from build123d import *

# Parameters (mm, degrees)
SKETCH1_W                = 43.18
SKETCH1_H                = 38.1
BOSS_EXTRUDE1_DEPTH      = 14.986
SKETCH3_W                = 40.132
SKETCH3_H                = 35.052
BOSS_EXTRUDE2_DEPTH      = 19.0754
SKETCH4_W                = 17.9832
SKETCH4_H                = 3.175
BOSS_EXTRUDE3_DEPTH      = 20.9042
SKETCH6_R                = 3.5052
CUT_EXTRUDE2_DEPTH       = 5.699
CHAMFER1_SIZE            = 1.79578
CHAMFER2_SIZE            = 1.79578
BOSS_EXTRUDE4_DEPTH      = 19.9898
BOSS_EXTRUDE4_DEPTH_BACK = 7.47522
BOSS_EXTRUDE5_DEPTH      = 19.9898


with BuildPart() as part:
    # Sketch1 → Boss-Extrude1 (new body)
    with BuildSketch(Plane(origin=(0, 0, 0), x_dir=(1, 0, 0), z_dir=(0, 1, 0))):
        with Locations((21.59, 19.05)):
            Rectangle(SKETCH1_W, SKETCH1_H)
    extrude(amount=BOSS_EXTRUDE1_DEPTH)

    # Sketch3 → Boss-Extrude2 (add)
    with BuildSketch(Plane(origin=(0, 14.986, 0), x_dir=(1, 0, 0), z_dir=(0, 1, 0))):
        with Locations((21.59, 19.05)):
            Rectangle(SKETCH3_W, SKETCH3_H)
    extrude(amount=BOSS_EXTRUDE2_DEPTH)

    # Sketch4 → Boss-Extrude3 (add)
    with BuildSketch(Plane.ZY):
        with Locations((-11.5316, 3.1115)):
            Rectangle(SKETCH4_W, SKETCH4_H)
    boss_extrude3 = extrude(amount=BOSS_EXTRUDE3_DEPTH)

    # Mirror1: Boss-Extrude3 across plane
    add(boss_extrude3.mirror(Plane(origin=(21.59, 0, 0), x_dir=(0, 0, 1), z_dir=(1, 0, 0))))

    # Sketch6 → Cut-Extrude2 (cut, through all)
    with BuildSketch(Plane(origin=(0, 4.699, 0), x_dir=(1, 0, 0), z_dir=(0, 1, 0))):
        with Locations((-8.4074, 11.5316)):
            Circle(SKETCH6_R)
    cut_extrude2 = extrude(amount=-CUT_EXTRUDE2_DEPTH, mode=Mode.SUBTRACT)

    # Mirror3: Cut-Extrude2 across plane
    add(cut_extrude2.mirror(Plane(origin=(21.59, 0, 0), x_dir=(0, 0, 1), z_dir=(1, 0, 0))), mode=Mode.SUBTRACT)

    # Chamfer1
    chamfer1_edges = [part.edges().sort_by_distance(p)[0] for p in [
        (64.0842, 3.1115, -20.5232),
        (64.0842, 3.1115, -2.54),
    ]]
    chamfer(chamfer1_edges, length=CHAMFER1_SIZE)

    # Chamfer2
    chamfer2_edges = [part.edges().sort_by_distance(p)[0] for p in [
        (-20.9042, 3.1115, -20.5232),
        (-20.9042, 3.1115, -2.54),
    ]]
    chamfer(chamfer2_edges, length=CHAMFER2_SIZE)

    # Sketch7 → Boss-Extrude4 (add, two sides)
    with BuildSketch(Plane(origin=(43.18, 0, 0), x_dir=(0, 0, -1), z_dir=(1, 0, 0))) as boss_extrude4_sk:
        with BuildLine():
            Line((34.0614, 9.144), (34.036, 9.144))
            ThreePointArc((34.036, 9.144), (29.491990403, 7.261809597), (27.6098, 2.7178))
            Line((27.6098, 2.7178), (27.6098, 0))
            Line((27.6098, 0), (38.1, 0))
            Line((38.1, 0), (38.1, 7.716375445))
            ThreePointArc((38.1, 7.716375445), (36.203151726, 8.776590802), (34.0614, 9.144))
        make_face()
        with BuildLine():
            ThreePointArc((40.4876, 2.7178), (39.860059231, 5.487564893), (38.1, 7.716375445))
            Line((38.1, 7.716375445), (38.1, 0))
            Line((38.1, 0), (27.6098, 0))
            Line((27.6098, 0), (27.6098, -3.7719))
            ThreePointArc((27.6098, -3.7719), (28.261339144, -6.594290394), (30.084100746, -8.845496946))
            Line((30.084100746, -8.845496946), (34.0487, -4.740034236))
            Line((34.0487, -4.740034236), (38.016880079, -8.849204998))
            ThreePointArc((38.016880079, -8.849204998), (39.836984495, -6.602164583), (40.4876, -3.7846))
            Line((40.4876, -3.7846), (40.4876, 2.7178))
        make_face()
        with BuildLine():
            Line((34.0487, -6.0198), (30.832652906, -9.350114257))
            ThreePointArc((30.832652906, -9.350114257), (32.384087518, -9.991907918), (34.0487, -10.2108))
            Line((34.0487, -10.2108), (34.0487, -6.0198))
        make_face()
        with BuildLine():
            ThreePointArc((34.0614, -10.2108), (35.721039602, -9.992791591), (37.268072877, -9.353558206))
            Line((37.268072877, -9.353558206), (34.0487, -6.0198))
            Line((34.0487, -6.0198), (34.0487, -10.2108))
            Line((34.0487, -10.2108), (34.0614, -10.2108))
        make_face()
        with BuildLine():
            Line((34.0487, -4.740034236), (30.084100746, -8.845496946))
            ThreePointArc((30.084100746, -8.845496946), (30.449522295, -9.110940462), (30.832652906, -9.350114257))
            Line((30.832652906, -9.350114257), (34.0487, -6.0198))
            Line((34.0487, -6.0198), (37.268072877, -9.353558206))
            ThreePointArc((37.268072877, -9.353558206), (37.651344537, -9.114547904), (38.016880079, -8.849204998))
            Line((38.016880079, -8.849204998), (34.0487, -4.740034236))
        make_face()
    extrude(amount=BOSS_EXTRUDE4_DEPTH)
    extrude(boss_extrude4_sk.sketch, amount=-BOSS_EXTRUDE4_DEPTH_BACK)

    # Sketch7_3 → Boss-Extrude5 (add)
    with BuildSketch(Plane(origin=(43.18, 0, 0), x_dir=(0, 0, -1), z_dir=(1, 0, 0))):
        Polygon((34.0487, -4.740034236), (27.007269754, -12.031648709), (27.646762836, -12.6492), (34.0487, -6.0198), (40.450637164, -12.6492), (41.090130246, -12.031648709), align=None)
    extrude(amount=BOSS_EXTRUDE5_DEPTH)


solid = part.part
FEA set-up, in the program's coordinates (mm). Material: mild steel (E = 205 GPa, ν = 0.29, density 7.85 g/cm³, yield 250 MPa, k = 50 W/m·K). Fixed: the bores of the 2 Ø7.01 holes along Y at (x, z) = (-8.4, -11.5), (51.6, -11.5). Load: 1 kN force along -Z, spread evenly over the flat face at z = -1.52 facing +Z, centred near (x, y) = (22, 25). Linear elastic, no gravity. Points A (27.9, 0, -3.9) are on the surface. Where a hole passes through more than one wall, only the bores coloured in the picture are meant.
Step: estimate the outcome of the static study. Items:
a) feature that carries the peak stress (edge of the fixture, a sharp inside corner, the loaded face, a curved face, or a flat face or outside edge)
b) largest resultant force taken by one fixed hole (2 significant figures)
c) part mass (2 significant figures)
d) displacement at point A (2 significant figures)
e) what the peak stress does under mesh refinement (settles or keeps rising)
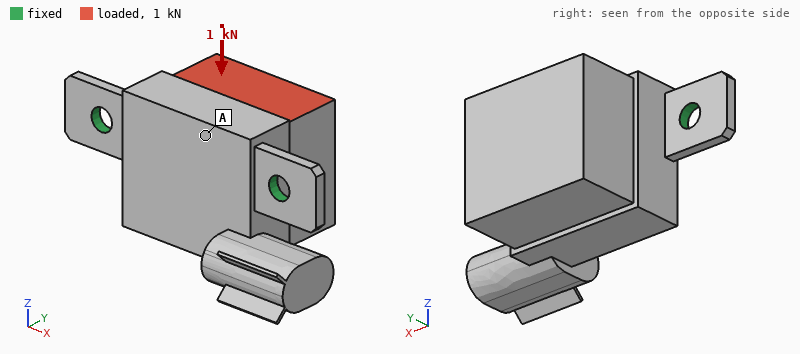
edge of the fixture
500 N
460 g
0.022 mm
keeps rising
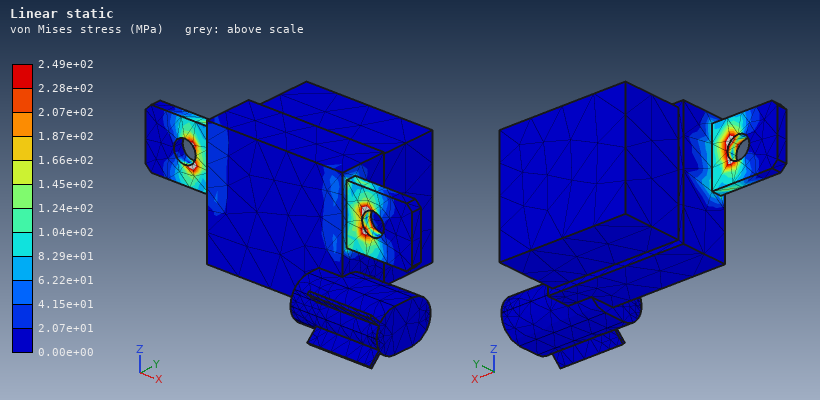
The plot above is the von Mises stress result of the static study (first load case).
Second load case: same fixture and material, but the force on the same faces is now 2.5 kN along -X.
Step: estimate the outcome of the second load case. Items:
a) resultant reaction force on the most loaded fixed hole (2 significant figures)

1.7 kN
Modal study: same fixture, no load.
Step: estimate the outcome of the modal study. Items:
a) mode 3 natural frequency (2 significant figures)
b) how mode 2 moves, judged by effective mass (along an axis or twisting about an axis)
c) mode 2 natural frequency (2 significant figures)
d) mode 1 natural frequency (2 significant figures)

4900 Hz
along Y
4500 Hz
990 Hz
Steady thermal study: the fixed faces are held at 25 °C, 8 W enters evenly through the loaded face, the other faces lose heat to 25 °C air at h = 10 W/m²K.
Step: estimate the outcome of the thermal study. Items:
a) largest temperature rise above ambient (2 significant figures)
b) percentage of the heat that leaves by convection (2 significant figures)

15 K
15 %
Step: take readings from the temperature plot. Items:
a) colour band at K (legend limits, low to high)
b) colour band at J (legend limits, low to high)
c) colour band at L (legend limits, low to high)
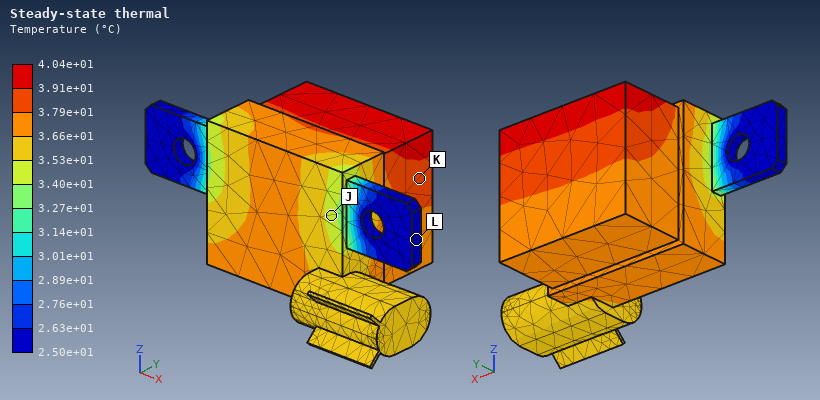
3.79e+01 to 3.91e+01 °C
3.40e+01 to 3.53e+01 °C
2.50e+01 to 2.63e+01 °C
